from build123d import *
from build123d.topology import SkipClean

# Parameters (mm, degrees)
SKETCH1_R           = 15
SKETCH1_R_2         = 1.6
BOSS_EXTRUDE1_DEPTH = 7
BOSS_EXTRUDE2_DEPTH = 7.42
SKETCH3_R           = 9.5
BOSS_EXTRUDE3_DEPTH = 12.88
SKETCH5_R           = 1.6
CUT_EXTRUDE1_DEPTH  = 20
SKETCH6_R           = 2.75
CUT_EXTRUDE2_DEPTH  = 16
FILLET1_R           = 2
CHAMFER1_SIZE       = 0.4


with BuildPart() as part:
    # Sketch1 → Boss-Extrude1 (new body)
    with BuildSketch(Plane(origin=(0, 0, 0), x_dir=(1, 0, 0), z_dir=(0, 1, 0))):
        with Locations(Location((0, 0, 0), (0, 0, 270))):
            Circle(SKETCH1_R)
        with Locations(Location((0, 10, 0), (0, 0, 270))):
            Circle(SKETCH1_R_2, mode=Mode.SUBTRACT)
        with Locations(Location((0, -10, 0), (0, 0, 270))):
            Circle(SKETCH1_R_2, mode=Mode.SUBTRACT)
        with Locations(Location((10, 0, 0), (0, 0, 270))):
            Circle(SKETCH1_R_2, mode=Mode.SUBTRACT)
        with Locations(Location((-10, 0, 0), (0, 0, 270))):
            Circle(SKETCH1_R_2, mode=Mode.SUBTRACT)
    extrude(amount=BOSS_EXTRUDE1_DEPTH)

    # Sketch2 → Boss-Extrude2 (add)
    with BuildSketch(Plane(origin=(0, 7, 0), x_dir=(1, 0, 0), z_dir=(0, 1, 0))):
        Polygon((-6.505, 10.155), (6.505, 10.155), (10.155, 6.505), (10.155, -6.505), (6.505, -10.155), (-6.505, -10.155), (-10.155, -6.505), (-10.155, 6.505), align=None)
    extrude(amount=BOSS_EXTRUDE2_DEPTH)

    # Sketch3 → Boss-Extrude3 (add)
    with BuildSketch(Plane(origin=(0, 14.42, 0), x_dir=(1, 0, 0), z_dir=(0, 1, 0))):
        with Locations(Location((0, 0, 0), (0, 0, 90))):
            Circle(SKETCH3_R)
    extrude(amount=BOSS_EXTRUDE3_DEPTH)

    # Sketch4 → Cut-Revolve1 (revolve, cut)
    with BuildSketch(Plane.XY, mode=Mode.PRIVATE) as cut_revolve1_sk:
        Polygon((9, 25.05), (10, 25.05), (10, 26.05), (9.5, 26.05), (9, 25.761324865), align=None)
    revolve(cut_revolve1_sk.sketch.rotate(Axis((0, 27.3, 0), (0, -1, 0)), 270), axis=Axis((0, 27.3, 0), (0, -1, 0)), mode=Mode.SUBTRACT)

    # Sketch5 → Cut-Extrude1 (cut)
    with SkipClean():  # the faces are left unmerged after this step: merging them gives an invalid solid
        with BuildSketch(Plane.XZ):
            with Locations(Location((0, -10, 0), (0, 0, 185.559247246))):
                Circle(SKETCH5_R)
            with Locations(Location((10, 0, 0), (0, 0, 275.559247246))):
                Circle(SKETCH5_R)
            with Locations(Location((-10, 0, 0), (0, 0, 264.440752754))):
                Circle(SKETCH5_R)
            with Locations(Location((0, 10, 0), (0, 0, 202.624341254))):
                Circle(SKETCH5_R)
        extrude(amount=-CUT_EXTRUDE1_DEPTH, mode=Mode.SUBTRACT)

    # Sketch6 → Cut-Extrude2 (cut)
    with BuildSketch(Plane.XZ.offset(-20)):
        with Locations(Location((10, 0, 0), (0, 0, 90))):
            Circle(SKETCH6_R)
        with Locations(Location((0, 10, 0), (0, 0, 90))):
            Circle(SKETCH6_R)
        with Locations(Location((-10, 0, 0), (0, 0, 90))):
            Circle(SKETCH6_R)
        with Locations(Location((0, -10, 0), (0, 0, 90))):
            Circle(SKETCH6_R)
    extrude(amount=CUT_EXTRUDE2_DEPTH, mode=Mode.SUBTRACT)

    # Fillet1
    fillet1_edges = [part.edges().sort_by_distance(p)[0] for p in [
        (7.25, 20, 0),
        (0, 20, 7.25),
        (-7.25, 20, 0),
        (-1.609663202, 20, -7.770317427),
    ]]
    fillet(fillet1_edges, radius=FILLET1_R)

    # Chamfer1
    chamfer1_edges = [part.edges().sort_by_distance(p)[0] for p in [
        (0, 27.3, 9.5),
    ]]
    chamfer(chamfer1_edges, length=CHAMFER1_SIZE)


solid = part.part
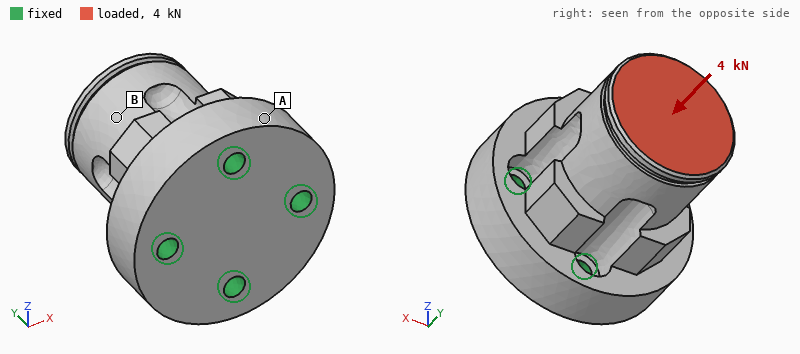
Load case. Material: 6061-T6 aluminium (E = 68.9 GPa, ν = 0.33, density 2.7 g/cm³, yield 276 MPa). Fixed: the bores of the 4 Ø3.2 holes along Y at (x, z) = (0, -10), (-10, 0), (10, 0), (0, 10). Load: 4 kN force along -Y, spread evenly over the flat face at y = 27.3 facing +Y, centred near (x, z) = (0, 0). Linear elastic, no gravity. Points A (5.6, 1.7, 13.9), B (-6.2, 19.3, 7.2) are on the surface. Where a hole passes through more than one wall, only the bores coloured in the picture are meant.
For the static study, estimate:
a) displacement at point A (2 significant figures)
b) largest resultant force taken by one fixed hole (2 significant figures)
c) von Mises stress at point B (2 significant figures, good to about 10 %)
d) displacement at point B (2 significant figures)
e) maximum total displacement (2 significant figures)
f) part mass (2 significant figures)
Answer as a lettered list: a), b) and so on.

a) 1.9 µm
b) 1.0 kN
c) 15 MPa
d) 5.5 µm
e) 7.3 µm
f) 28 g
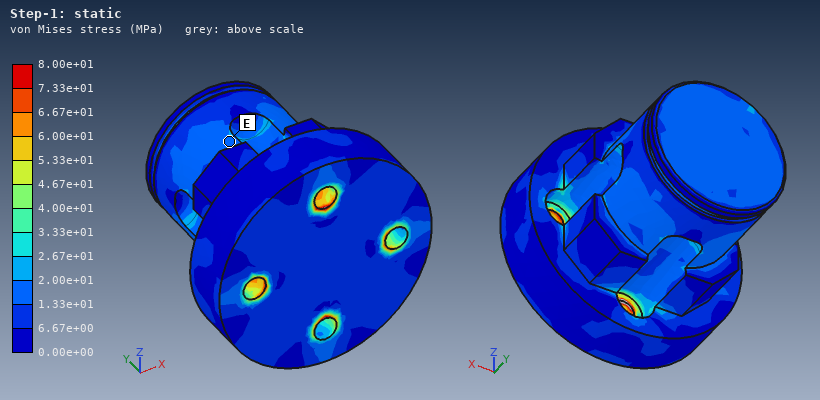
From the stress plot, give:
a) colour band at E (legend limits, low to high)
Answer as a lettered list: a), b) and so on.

a) 1.33e+01 to 2.00e+01 MPa
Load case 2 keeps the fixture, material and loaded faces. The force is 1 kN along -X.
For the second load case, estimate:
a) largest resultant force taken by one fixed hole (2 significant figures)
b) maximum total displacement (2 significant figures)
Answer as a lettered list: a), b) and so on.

a) 1.2 kN
b) 20 µm
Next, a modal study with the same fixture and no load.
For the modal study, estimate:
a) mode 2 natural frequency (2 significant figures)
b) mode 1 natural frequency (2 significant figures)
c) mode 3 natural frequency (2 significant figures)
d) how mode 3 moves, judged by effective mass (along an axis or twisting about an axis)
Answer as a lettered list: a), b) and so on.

a) 15 kHz
b) 15 kHz
c) 31 kHz
d) twisting about Y
